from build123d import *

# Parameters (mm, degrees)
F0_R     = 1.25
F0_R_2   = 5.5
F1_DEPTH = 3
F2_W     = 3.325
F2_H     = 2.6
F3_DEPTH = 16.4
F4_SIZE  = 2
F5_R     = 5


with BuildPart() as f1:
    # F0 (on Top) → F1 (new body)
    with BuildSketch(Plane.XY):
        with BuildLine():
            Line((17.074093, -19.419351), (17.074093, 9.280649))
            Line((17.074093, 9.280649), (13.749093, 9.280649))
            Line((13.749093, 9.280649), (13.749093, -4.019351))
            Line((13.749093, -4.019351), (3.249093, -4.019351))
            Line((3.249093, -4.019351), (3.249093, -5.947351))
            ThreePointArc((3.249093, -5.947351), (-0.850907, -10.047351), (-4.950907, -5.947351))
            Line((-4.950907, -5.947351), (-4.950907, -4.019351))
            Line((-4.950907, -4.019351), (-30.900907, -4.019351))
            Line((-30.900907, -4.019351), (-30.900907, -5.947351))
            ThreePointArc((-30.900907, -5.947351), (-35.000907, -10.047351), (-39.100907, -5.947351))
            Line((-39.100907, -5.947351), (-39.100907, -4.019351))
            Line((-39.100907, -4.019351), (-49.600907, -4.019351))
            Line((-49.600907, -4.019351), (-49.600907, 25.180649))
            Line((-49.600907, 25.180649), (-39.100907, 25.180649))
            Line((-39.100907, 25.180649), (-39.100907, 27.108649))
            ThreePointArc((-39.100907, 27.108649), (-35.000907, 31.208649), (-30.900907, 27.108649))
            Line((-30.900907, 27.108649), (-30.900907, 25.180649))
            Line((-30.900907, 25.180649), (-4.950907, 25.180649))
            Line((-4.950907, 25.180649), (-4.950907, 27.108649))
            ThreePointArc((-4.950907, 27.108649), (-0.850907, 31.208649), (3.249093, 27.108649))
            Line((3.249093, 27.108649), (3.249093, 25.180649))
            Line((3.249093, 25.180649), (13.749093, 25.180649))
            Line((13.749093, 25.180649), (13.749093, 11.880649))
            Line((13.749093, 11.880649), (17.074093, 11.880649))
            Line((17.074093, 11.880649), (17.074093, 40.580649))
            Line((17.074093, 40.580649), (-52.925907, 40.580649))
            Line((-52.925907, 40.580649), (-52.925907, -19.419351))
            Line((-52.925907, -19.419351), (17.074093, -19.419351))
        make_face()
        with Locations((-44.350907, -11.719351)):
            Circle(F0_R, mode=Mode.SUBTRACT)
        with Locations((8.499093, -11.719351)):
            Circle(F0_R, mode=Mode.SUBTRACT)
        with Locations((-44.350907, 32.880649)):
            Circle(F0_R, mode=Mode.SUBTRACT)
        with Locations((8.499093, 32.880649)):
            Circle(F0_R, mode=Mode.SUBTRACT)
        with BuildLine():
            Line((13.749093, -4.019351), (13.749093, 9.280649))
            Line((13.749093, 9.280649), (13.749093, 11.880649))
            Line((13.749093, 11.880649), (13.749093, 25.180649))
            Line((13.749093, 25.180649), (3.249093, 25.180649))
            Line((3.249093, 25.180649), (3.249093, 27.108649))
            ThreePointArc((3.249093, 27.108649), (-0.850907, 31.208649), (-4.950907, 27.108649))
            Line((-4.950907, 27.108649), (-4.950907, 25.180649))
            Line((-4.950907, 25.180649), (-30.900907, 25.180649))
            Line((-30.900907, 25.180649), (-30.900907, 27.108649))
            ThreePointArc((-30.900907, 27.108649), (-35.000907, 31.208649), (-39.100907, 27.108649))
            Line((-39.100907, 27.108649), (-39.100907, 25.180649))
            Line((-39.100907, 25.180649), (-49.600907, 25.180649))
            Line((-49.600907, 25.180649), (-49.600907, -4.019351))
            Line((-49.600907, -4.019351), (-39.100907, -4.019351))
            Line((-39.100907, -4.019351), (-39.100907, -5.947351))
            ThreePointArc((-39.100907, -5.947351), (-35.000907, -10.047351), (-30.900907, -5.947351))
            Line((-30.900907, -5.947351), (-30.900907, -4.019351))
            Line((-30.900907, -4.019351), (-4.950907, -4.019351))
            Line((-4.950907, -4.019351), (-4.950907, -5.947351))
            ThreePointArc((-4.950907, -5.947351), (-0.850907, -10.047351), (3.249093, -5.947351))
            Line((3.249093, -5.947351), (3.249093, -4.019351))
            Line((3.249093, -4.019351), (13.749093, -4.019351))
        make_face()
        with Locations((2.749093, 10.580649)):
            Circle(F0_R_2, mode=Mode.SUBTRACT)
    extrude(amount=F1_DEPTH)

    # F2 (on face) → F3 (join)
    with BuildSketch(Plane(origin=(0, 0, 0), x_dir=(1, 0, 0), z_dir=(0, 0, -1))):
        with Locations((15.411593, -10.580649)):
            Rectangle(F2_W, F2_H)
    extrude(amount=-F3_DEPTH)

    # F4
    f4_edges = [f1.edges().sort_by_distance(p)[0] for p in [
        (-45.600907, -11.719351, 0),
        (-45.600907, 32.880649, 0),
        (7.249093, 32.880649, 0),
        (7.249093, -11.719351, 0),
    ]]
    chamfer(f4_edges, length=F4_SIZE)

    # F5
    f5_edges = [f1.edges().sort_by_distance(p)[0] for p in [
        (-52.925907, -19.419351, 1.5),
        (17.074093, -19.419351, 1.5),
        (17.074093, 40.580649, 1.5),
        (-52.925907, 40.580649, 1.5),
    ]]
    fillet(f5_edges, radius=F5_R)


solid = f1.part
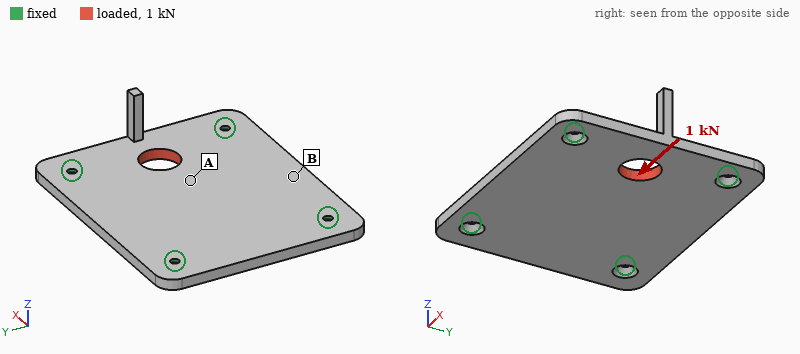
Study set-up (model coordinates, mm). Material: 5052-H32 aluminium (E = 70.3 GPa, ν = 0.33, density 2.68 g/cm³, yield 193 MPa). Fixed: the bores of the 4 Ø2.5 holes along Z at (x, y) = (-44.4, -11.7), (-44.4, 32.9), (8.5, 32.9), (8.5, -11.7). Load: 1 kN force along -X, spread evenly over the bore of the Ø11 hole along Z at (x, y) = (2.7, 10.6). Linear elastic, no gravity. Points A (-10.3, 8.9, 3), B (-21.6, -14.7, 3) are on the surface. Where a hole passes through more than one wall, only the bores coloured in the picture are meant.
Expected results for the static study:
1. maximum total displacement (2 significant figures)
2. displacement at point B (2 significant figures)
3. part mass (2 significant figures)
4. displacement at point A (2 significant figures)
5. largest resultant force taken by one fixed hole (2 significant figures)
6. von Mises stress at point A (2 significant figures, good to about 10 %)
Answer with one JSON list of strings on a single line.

["7.5 µm", "2.1 µm", "33 g", "4.1 µm", "290 N", "7.5 MPa"]
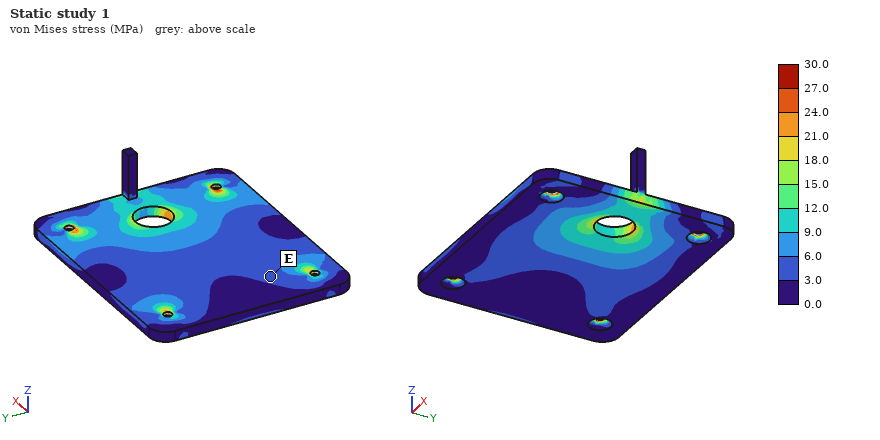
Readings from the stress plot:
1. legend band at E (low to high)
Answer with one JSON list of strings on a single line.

["3.0 to 6.0 MPa"]
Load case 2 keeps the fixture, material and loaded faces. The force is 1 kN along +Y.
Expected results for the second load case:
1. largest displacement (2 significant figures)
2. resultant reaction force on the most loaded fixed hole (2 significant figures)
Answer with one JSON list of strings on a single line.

["7.5 µm", "410 N"]
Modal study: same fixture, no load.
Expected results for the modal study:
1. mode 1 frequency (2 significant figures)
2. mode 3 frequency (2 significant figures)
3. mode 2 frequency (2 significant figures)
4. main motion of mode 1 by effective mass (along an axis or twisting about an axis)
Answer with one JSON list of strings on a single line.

["3400 Hz", "5200 Hz", "5000 Hz", "along Z"]
